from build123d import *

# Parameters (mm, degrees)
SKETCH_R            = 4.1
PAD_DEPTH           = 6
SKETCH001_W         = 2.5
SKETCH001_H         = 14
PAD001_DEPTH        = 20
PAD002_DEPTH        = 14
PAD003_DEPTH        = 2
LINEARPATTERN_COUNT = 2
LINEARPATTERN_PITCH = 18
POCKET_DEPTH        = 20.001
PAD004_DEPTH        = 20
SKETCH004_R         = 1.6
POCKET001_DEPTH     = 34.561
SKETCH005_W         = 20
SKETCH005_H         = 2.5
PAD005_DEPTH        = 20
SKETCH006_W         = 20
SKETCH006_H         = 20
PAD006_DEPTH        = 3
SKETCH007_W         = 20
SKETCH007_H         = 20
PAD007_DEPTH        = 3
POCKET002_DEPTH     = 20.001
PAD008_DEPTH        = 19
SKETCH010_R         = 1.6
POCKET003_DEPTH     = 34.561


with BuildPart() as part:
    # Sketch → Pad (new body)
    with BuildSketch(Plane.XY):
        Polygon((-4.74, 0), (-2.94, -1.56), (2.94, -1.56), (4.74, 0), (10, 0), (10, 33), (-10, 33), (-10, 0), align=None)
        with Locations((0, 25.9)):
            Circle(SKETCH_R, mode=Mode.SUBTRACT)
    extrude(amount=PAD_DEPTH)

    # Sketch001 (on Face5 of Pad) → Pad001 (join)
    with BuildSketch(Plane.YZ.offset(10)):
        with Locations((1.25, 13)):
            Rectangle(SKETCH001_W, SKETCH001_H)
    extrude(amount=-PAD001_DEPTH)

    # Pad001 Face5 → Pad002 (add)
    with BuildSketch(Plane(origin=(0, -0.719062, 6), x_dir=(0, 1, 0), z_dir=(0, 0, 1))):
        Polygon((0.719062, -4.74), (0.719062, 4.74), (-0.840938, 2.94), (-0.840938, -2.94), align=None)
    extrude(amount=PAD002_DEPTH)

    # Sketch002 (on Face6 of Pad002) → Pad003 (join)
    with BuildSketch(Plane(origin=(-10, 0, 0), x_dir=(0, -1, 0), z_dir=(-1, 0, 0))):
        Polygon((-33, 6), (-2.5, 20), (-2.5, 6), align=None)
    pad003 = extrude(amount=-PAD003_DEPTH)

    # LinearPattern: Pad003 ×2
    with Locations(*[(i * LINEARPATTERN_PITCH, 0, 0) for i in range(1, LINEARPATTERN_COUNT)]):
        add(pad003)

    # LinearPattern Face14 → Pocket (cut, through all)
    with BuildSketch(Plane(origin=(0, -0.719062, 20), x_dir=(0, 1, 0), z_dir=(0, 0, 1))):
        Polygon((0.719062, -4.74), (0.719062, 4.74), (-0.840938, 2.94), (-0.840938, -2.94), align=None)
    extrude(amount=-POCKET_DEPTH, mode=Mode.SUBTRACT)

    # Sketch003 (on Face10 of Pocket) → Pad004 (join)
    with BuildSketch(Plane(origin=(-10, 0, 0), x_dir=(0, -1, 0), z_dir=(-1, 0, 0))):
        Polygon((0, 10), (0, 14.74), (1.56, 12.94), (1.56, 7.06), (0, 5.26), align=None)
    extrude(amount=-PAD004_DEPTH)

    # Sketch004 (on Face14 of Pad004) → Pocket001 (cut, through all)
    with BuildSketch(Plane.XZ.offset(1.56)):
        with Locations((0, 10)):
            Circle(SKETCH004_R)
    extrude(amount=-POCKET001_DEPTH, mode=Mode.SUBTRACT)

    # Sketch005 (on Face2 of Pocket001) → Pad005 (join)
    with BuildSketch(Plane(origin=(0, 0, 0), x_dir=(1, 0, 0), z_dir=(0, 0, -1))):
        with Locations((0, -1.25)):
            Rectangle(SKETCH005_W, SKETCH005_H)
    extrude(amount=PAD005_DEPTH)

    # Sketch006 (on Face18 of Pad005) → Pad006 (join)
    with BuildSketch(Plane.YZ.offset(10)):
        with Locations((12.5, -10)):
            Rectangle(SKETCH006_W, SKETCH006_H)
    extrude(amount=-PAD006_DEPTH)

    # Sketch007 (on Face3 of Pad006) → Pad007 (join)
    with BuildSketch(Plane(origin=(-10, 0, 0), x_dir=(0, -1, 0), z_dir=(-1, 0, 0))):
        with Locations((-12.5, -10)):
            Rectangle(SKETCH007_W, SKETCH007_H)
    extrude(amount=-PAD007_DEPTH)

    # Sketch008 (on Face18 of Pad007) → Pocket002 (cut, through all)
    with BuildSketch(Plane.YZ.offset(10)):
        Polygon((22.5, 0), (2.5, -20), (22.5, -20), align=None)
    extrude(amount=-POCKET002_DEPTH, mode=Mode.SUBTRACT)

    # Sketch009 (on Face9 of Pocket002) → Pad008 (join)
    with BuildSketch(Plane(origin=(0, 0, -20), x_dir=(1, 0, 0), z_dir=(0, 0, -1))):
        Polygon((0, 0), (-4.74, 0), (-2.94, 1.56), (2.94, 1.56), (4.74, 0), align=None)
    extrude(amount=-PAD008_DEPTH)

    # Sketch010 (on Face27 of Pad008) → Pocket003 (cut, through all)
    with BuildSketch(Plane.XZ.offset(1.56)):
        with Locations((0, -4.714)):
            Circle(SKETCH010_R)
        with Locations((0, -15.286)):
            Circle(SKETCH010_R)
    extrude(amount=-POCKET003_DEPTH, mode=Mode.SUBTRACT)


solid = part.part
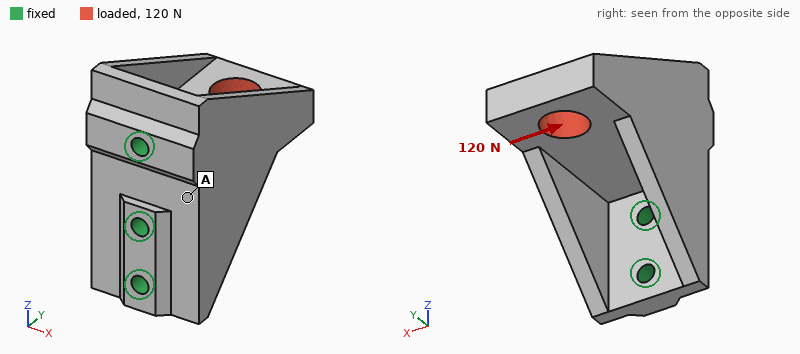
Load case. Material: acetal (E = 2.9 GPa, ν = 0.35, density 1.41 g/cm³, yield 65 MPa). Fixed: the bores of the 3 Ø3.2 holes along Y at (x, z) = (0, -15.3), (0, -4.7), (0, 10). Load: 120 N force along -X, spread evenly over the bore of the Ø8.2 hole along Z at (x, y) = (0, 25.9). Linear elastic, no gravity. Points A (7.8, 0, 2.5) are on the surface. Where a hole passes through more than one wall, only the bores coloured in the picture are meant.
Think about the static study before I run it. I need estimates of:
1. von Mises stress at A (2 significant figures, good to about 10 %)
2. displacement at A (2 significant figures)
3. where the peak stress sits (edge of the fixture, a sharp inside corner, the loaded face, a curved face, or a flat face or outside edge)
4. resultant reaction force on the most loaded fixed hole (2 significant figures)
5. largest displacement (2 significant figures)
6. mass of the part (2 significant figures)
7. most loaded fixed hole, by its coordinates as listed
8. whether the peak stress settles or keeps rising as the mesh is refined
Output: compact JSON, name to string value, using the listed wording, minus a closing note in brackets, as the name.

{"von Mises stress at A": "5.1 MPa", "displacement at A": "0.10 mm", "where the peak stress sits": "edge of the fixture", "resultant reaction force on the most loaded fixed hole": "100 N", "largest displacement": "0.52 mm", "mass of the part": "11 g", "most loaded fixed hole, by its coordinates as listed": "(0, -4.7)", "whether the peak stress settles or keeps rising as the mesh is refined": "keeps rising"}
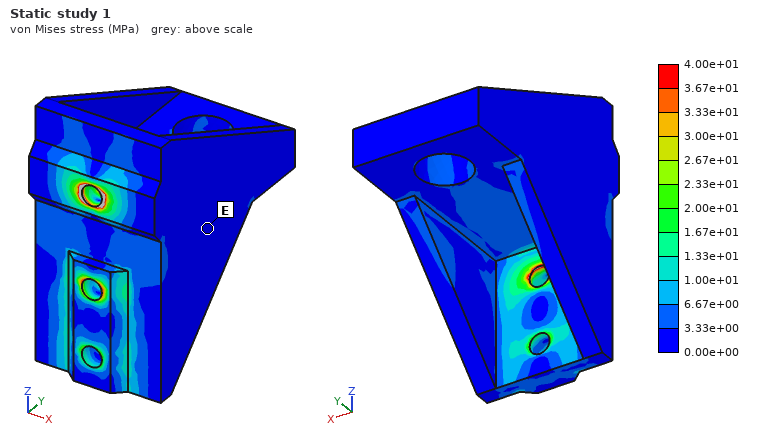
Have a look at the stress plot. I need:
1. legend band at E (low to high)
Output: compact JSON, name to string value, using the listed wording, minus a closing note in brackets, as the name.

{"legend band at E": "0.00e+00 to 3.33e+00 MPa"}
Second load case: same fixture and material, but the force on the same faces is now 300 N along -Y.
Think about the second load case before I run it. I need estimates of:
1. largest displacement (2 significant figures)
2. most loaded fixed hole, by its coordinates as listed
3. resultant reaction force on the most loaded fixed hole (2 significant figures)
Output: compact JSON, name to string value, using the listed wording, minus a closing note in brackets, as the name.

{"largest displacement": "62 µm", "most loaded fixed hole, by its coordinates as listed": "(0, 10)", "resultant reaction force on the most loaded fixed hole": "180 N"}
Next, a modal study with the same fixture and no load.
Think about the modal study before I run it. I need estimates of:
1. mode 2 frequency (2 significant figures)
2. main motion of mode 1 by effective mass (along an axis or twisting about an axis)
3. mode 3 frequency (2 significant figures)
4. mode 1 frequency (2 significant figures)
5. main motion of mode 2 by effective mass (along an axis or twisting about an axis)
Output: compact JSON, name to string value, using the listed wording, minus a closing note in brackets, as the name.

{"mode 2 frequency": "2600 Hz", "main motion of mode 1 by effective mass": "along X", "mode 3 frequency": "4200 Hz", "mode 1 frequency": "1500 Hz", "main motion of mode 2 by effective mass": "along Z"}
